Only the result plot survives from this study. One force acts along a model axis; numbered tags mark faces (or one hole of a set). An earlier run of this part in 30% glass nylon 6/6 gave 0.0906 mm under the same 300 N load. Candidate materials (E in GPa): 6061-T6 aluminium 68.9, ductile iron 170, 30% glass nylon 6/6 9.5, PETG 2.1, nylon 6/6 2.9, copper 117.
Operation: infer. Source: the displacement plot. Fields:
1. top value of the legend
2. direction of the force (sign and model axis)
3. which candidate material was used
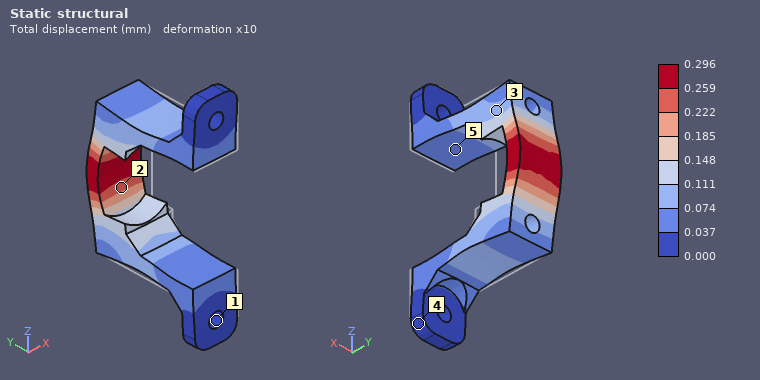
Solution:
0.296 mm
+Y
nylon 6/6
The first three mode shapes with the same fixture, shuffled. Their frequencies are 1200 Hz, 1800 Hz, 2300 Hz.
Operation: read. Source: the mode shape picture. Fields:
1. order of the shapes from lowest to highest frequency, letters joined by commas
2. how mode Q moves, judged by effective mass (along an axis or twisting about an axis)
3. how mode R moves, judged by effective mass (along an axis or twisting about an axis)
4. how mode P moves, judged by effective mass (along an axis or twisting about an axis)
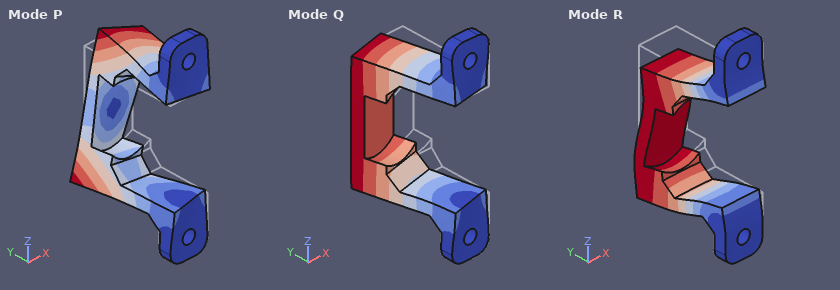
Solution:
Q, R, P
along X
along Z
twisting about Y
